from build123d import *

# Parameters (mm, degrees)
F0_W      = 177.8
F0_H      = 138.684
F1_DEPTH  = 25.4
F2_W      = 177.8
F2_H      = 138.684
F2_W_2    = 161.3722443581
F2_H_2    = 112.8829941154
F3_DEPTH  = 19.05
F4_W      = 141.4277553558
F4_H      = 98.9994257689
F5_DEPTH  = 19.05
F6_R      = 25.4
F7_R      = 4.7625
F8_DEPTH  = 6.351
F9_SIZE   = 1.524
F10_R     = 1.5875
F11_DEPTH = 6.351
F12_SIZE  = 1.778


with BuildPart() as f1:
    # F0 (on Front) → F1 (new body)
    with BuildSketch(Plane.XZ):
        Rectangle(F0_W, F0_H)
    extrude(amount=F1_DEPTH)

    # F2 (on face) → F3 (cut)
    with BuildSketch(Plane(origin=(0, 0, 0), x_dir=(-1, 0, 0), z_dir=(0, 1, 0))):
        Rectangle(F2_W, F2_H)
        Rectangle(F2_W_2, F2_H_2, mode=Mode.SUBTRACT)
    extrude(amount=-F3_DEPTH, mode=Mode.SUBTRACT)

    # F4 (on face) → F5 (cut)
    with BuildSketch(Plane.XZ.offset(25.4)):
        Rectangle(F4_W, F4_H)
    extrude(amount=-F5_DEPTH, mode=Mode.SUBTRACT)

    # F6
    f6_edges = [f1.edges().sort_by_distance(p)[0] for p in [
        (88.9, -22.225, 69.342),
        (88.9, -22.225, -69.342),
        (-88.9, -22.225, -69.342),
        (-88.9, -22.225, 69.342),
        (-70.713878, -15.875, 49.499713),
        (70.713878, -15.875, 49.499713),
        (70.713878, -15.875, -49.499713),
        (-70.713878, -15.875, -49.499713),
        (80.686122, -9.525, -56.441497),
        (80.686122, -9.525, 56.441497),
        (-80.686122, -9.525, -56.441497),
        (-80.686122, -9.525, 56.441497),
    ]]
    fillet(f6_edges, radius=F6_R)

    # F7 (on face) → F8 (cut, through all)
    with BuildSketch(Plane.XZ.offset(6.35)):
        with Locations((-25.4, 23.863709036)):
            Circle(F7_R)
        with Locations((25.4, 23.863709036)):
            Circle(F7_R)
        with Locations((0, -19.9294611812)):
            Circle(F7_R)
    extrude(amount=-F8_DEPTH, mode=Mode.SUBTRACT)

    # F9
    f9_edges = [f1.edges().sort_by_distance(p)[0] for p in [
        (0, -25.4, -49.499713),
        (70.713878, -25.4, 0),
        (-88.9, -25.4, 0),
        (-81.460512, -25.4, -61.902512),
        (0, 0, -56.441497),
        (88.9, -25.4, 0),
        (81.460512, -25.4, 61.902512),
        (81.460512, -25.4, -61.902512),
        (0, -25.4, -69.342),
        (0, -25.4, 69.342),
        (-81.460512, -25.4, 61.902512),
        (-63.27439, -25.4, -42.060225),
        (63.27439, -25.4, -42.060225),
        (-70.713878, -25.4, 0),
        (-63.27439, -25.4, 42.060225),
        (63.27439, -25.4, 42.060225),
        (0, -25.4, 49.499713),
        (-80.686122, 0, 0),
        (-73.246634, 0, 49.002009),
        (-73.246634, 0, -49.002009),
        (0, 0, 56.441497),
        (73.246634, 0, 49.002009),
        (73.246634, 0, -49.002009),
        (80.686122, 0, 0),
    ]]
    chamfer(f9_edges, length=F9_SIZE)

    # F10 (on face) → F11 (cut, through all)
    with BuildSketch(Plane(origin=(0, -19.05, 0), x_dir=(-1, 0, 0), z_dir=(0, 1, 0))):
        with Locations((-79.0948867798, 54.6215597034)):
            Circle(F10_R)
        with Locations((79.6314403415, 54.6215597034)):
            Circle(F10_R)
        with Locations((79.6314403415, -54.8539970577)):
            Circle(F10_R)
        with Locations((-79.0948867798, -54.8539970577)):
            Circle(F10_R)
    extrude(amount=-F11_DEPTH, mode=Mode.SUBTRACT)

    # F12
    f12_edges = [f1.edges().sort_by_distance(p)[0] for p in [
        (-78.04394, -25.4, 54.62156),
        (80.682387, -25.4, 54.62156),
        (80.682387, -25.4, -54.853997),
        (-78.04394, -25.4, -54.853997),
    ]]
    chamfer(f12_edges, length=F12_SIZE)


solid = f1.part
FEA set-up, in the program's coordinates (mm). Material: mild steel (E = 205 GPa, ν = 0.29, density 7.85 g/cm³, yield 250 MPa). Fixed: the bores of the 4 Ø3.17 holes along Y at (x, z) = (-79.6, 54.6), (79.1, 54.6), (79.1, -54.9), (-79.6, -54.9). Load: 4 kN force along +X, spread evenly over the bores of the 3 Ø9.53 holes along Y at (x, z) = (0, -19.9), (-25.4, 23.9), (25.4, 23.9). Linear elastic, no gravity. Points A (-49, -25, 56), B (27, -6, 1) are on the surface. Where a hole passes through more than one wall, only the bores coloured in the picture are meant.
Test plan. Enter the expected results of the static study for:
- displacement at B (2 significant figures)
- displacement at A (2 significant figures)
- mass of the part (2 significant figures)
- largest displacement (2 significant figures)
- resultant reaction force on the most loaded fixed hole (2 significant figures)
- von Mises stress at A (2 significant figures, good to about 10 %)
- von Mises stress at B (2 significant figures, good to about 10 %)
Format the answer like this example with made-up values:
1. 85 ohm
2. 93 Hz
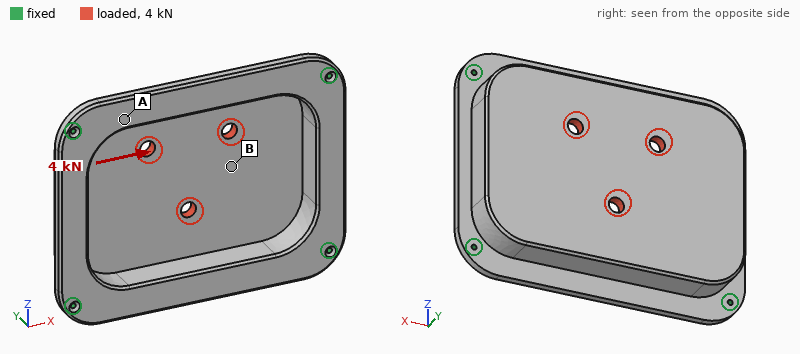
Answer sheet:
1. 2.8 µm
2. 1.2 µm
3. 1.8 kg
4. 3.3 µm
5. 1.1 kN
6. 5.0 MPa
7. 1.7 MPa
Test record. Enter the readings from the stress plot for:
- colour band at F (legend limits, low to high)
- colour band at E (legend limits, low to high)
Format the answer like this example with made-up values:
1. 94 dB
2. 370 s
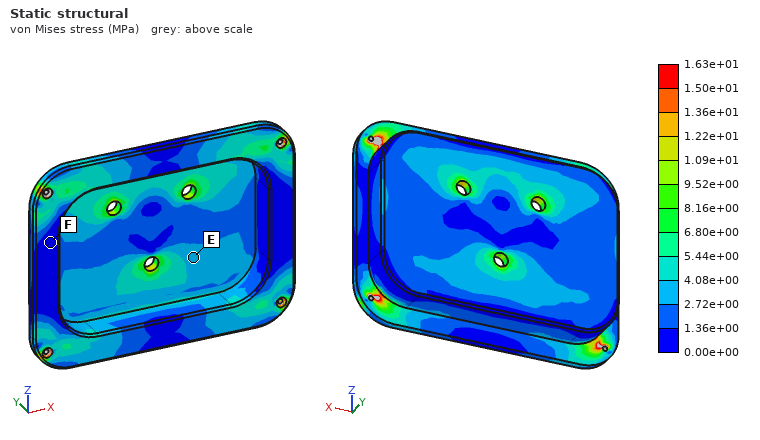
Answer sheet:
1. 0.00e+00 to 1.36e+00 MPa
2. 2.72e+00 to 4.08e+00 MPa
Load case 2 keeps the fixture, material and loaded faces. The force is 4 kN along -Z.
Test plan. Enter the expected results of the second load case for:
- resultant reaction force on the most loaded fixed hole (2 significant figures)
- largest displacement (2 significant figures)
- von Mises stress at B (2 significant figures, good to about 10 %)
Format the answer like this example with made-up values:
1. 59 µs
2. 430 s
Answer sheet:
1. 1.1 kN
2. 5.6 µm
3. 6.1 MPa
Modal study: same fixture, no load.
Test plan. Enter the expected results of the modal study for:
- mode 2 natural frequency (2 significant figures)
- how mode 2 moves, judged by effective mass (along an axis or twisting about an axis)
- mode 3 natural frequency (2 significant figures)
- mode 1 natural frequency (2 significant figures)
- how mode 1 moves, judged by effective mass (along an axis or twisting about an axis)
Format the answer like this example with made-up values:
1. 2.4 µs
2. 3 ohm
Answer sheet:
1. 2700 Hz
2. twisting about X
3. 3300 Hz
4. 2300 Hz
5. along Y
